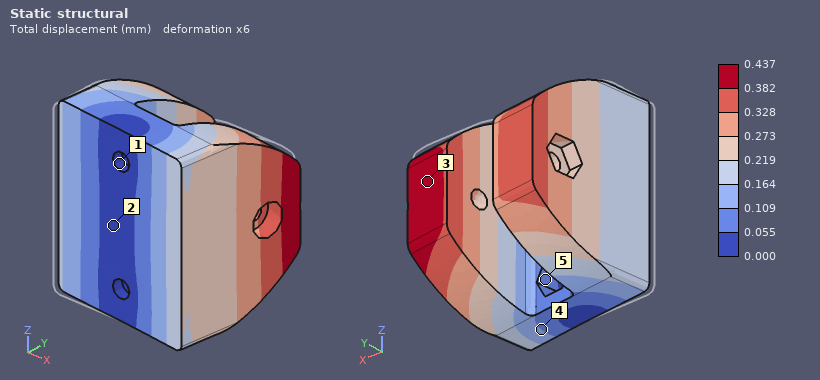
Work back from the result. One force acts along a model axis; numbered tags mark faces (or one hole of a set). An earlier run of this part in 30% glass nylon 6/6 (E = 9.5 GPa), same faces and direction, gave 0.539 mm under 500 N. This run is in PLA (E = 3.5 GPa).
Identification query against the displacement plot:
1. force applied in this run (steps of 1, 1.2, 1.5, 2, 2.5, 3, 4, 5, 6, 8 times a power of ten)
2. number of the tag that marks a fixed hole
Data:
150 N
1
